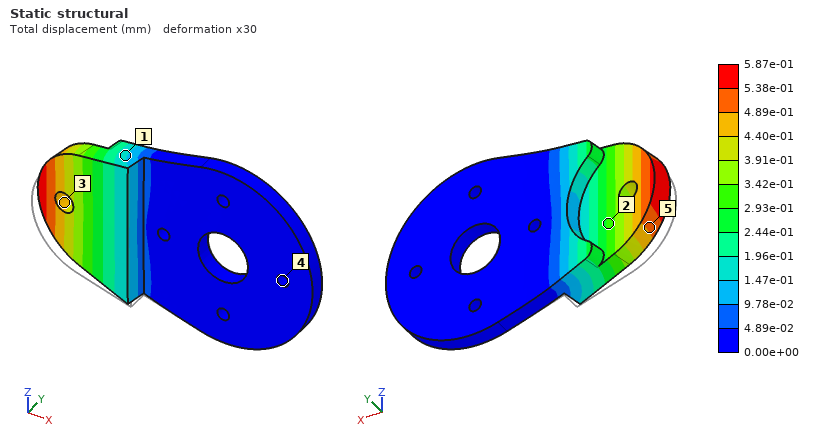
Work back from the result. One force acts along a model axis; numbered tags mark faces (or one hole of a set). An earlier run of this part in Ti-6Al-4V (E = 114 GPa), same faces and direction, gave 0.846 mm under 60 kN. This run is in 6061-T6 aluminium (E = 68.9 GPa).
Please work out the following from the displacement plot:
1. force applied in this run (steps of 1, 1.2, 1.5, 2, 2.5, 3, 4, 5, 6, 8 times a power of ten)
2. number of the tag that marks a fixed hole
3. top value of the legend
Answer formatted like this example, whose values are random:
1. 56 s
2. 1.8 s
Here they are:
1. 25 kN
2. 4
3. 5.87e-01 mm
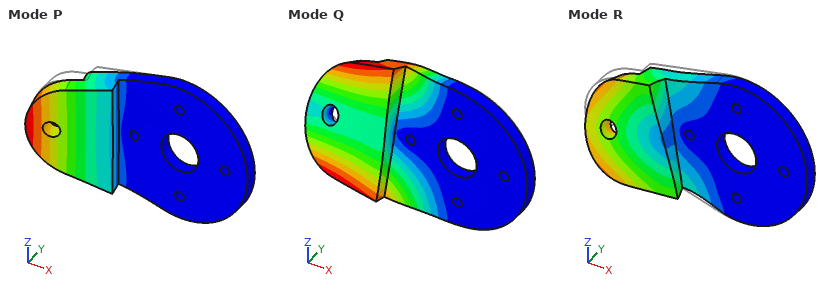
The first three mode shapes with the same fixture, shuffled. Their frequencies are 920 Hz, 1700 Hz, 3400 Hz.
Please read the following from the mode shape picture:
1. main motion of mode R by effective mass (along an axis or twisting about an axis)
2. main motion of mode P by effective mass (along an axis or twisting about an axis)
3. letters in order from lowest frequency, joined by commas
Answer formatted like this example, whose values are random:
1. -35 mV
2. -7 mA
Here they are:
1. along Z
2. along Y
3. P, Q, R
